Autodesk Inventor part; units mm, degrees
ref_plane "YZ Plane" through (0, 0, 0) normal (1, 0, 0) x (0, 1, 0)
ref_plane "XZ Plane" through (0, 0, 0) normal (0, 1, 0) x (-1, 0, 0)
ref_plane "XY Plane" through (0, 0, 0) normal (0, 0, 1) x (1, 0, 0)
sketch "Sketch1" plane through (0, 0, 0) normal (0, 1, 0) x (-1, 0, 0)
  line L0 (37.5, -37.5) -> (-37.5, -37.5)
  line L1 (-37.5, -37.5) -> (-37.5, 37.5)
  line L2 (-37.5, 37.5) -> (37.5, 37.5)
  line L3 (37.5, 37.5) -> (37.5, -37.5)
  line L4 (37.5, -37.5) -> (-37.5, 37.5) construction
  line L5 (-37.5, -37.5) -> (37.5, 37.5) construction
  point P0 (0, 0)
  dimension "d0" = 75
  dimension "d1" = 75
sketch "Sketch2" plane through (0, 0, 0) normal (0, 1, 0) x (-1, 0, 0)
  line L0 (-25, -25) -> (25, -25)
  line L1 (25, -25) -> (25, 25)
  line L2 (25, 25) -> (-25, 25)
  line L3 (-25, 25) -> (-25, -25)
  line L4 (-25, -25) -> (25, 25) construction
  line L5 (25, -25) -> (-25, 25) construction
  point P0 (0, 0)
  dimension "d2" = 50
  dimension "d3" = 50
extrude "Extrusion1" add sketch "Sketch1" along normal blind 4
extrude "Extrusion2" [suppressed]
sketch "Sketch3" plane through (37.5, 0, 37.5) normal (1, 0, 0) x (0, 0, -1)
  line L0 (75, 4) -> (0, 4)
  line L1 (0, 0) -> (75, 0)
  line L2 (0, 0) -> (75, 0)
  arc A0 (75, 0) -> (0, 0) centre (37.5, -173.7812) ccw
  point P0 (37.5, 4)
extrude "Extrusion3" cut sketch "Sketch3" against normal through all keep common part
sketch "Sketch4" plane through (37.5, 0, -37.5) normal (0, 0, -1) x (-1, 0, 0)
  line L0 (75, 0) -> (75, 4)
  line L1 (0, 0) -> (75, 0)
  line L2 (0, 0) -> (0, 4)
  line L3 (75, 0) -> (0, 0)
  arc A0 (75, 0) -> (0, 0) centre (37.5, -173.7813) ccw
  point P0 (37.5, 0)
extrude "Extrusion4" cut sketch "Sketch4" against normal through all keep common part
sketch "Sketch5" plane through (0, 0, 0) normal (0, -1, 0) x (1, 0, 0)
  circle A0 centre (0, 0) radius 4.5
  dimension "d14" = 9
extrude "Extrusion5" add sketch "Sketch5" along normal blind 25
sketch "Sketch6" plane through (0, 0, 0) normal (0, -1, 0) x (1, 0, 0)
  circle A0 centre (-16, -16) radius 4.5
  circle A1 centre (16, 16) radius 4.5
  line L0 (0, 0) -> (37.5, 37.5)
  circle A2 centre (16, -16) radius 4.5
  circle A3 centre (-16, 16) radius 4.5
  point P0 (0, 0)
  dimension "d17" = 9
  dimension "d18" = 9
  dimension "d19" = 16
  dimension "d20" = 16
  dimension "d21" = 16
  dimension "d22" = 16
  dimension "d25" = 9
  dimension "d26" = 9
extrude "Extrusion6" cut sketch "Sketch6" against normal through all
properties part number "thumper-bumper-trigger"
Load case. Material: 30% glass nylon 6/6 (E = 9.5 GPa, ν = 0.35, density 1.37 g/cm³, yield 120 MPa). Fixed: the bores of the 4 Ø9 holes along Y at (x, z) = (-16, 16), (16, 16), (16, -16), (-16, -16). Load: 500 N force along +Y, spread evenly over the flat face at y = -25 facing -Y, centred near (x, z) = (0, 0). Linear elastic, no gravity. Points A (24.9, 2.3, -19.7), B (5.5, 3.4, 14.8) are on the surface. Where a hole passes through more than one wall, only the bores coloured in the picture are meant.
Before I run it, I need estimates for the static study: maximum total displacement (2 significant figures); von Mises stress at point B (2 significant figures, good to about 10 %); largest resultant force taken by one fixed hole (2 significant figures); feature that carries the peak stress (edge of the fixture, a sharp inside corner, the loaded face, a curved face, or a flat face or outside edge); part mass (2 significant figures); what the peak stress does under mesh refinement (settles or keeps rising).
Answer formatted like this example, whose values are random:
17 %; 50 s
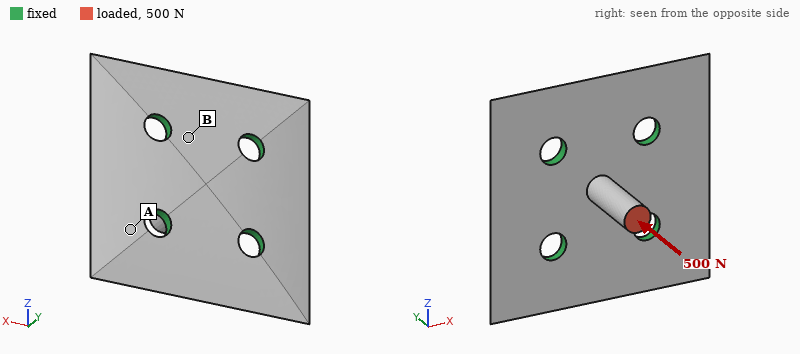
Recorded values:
97 µm; 7.1 MPa; 130 N; edge of the fixture; 17 g; keeps rising
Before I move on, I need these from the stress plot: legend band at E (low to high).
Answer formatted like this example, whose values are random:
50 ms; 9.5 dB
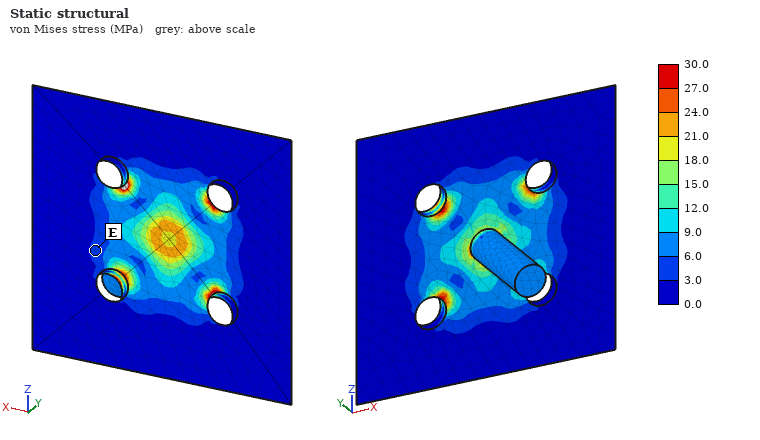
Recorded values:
3.0 to 6.0 MPa
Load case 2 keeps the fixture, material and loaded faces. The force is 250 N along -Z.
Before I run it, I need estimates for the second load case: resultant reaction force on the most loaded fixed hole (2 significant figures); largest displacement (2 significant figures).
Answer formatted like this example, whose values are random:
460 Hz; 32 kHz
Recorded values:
160 N; 0.84 mm
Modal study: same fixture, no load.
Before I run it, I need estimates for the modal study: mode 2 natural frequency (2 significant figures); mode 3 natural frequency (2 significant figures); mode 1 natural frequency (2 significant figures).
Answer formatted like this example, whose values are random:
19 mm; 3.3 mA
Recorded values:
3400 Hz; 3600 Hz; 3400 Hz
